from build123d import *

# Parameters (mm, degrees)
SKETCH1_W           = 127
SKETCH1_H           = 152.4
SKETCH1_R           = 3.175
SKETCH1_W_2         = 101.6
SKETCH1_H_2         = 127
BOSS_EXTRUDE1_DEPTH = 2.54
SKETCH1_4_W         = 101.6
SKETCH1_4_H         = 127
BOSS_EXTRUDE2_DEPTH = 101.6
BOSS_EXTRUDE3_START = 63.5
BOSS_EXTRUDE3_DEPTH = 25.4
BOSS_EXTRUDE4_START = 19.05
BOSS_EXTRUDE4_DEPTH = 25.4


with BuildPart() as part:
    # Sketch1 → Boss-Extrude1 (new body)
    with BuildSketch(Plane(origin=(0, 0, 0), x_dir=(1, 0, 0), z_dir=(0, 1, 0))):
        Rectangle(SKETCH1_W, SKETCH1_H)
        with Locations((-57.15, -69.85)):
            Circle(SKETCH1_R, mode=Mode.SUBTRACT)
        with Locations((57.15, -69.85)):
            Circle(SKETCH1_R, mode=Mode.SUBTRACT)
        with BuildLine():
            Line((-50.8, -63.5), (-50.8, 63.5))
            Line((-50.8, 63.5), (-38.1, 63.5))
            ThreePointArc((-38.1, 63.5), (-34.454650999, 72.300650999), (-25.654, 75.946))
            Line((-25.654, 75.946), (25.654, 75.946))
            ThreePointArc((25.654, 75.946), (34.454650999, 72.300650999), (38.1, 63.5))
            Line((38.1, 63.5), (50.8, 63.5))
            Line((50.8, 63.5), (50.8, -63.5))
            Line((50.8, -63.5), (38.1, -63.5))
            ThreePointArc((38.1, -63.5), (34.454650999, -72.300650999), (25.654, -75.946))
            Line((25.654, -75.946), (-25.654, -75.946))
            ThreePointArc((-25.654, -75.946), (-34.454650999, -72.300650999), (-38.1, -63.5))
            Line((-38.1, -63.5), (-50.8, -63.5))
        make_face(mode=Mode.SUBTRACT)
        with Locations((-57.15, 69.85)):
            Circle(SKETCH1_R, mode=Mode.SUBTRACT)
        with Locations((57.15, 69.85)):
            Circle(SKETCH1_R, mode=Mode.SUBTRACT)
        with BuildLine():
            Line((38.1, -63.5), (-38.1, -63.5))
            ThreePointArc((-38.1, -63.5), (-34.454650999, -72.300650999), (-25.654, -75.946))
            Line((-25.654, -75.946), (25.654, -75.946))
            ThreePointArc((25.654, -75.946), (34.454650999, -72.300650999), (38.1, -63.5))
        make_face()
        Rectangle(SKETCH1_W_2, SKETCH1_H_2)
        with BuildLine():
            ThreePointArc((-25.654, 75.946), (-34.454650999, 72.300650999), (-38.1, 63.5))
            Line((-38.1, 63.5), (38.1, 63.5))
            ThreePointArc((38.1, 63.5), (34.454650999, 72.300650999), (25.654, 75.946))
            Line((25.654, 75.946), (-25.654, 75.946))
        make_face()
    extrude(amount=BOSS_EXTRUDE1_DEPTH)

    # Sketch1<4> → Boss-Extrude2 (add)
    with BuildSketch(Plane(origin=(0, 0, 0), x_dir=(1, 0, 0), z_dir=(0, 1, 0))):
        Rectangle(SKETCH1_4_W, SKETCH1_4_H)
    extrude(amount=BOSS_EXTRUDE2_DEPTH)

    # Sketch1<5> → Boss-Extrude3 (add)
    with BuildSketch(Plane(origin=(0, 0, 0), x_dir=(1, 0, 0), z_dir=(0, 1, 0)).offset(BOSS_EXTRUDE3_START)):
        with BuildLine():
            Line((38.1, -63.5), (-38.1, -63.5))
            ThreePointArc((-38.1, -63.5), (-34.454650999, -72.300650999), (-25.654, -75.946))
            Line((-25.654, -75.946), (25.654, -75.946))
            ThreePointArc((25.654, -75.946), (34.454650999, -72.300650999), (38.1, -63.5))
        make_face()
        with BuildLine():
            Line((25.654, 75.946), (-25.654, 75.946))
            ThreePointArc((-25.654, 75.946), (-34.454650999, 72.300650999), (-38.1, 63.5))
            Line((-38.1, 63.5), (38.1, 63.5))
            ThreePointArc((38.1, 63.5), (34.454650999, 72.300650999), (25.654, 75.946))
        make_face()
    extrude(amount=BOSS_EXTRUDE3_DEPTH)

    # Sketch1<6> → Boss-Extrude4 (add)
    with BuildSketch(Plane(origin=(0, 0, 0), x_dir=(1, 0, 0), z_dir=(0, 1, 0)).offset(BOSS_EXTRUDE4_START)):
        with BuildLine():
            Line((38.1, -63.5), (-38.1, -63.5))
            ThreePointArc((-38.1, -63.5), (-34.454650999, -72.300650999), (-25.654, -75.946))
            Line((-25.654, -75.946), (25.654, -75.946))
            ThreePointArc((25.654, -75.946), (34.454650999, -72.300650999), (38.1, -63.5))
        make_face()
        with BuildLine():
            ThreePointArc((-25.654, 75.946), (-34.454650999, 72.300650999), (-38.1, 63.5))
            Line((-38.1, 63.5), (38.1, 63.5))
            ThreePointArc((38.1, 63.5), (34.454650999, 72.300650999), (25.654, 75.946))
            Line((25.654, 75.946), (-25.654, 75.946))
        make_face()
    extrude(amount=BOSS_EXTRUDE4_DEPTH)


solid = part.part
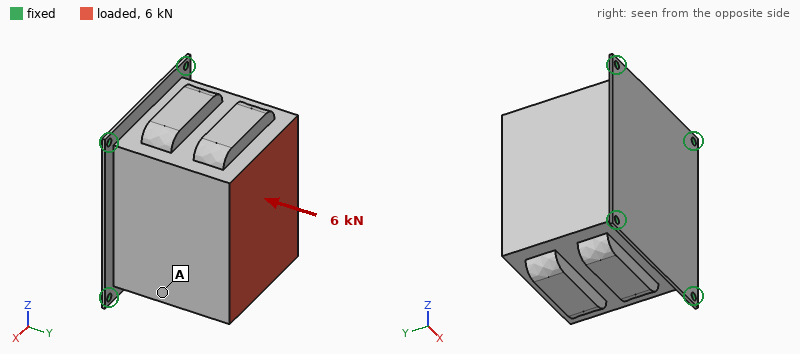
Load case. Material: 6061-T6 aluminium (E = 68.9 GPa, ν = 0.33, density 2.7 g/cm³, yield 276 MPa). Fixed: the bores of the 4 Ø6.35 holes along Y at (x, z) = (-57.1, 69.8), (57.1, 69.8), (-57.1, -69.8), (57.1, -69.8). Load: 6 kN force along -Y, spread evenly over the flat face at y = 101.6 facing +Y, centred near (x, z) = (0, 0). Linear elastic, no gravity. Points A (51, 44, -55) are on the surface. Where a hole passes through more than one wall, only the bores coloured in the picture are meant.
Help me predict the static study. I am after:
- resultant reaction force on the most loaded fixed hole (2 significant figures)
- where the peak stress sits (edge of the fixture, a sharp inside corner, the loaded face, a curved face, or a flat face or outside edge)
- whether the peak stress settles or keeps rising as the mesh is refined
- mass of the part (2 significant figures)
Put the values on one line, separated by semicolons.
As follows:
1.7 kN; edge of the fixture; keeps rising; 3.8 kg
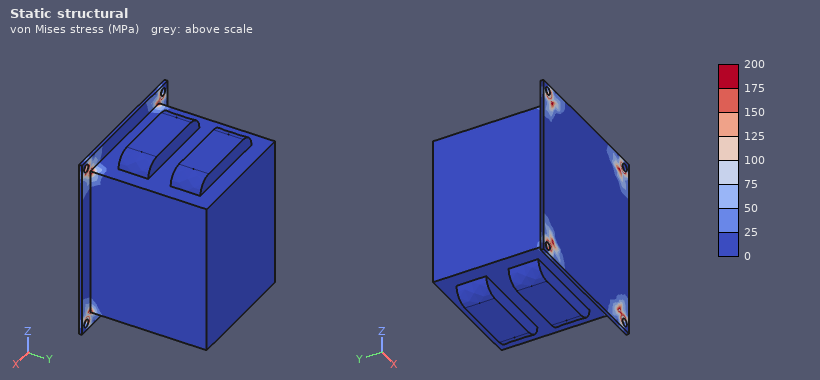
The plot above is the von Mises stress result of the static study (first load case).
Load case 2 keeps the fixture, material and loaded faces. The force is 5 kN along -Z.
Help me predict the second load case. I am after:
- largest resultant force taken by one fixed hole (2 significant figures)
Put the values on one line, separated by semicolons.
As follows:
2.5 kN
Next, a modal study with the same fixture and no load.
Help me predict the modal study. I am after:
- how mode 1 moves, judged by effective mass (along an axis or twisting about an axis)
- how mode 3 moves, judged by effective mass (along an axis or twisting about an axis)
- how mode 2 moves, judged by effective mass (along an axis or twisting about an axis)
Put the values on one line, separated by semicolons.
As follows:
along X; along Y; along Z
